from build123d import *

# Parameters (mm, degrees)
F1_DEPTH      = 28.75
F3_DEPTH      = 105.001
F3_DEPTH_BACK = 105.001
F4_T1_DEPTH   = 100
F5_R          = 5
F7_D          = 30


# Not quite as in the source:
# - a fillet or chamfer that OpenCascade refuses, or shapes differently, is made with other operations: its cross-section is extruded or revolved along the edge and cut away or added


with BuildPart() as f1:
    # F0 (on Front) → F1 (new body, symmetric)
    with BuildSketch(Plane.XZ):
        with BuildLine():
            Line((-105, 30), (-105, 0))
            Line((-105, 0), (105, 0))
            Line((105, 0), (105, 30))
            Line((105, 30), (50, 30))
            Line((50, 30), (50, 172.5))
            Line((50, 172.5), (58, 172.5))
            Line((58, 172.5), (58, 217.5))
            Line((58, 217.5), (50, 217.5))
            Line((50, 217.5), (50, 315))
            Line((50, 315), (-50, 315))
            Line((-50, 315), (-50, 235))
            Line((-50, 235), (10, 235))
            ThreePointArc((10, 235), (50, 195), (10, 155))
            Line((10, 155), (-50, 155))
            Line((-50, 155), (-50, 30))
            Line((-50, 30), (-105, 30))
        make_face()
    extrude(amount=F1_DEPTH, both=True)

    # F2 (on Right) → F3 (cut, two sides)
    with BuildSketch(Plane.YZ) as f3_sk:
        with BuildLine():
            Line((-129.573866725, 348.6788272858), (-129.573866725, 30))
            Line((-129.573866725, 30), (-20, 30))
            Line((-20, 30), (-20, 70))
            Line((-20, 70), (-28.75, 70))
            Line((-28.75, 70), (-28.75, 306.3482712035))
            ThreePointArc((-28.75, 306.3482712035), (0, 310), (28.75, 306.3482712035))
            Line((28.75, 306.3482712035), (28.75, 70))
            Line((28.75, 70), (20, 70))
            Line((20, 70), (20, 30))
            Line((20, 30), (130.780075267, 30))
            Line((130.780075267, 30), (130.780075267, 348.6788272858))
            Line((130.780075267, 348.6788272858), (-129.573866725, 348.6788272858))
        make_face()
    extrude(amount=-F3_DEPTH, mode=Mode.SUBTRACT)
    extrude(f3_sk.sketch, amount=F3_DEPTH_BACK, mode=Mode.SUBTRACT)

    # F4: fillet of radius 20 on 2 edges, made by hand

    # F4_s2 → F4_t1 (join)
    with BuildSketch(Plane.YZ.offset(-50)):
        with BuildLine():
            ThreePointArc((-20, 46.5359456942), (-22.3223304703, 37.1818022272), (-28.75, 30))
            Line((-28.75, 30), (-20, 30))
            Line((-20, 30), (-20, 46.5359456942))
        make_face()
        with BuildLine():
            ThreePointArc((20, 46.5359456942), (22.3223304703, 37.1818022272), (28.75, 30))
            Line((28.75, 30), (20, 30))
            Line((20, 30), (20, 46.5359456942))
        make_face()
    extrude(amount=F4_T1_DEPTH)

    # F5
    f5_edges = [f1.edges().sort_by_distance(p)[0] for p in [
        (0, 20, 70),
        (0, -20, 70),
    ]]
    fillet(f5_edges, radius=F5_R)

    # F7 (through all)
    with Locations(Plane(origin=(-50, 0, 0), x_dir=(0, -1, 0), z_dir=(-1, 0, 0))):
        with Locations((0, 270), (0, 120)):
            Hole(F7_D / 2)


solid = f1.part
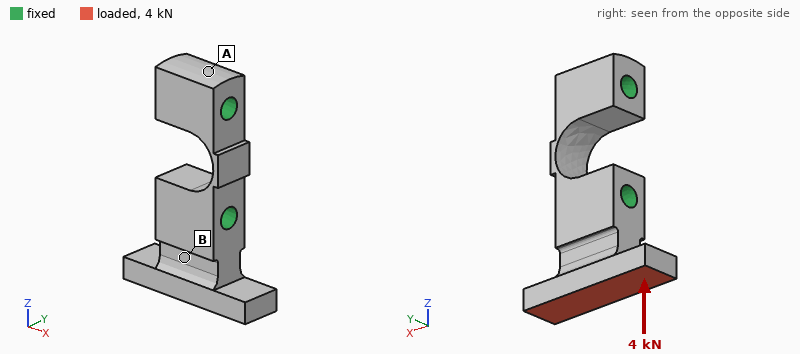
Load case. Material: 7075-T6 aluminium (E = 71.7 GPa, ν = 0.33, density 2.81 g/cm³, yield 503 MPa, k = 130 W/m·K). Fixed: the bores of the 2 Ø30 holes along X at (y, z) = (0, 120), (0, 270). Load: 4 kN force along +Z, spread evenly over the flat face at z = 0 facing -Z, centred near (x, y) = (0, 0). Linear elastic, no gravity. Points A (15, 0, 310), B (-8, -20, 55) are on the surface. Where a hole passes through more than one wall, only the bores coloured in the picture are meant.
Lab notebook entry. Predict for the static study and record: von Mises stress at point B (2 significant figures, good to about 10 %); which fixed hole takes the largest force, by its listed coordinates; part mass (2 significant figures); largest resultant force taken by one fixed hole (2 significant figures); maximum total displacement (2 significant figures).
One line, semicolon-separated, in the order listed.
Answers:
0.64 MPa; (0, 120); 3.8 kg; 4.0 kN; 9.3 µm
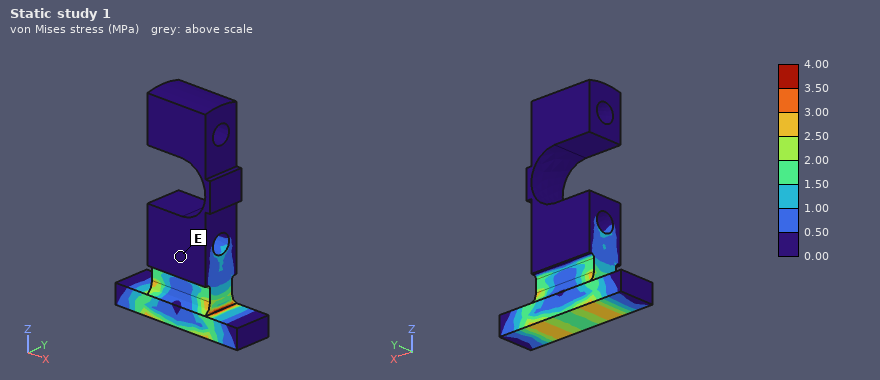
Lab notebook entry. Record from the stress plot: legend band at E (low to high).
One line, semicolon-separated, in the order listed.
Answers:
0.00 to 0.50 MPa
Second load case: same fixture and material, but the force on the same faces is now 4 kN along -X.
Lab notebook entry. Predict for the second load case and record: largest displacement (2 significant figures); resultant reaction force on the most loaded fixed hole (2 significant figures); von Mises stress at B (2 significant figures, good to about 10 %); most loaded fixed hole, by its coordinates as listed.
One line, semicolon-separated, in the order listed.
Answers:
18 µm; 4.0 kN; 2.8 MPa; (0, 120)
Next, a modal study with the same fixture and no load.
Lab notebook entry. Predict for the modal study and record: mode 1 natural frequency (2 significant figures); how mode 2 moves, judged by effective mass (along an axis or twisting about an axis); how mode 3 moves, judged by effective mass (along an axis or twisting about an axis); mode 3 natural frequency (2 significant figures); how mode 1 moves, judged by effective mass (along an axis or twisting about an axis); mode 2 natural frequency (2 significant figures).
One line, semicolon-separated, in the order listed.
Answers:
1900 Hz; twisting about Z; along X; 2700 Hz; along Y; 2200 Hz
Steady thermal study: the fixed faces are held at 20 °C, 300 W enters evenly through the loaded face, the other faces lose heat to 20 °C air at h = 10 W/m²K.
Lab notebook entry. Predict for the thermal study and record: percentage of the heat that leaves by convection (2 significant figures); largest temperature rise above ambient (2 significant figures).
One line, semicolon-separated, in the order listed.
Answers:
5.2 %; 57 K
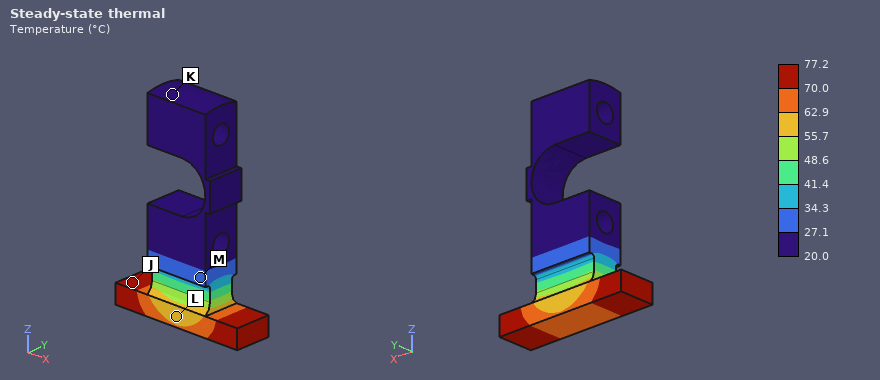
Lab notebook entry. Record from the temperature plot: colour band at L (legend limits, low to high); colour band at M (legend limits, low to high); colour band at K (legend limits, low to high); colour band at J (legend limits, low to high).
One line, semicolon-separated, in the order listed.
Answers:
55.7 to 62.9 °C; 27.1 to 34.3 °C; 20.0 to 27.1 °C; 70.0 to 77.2 °C
